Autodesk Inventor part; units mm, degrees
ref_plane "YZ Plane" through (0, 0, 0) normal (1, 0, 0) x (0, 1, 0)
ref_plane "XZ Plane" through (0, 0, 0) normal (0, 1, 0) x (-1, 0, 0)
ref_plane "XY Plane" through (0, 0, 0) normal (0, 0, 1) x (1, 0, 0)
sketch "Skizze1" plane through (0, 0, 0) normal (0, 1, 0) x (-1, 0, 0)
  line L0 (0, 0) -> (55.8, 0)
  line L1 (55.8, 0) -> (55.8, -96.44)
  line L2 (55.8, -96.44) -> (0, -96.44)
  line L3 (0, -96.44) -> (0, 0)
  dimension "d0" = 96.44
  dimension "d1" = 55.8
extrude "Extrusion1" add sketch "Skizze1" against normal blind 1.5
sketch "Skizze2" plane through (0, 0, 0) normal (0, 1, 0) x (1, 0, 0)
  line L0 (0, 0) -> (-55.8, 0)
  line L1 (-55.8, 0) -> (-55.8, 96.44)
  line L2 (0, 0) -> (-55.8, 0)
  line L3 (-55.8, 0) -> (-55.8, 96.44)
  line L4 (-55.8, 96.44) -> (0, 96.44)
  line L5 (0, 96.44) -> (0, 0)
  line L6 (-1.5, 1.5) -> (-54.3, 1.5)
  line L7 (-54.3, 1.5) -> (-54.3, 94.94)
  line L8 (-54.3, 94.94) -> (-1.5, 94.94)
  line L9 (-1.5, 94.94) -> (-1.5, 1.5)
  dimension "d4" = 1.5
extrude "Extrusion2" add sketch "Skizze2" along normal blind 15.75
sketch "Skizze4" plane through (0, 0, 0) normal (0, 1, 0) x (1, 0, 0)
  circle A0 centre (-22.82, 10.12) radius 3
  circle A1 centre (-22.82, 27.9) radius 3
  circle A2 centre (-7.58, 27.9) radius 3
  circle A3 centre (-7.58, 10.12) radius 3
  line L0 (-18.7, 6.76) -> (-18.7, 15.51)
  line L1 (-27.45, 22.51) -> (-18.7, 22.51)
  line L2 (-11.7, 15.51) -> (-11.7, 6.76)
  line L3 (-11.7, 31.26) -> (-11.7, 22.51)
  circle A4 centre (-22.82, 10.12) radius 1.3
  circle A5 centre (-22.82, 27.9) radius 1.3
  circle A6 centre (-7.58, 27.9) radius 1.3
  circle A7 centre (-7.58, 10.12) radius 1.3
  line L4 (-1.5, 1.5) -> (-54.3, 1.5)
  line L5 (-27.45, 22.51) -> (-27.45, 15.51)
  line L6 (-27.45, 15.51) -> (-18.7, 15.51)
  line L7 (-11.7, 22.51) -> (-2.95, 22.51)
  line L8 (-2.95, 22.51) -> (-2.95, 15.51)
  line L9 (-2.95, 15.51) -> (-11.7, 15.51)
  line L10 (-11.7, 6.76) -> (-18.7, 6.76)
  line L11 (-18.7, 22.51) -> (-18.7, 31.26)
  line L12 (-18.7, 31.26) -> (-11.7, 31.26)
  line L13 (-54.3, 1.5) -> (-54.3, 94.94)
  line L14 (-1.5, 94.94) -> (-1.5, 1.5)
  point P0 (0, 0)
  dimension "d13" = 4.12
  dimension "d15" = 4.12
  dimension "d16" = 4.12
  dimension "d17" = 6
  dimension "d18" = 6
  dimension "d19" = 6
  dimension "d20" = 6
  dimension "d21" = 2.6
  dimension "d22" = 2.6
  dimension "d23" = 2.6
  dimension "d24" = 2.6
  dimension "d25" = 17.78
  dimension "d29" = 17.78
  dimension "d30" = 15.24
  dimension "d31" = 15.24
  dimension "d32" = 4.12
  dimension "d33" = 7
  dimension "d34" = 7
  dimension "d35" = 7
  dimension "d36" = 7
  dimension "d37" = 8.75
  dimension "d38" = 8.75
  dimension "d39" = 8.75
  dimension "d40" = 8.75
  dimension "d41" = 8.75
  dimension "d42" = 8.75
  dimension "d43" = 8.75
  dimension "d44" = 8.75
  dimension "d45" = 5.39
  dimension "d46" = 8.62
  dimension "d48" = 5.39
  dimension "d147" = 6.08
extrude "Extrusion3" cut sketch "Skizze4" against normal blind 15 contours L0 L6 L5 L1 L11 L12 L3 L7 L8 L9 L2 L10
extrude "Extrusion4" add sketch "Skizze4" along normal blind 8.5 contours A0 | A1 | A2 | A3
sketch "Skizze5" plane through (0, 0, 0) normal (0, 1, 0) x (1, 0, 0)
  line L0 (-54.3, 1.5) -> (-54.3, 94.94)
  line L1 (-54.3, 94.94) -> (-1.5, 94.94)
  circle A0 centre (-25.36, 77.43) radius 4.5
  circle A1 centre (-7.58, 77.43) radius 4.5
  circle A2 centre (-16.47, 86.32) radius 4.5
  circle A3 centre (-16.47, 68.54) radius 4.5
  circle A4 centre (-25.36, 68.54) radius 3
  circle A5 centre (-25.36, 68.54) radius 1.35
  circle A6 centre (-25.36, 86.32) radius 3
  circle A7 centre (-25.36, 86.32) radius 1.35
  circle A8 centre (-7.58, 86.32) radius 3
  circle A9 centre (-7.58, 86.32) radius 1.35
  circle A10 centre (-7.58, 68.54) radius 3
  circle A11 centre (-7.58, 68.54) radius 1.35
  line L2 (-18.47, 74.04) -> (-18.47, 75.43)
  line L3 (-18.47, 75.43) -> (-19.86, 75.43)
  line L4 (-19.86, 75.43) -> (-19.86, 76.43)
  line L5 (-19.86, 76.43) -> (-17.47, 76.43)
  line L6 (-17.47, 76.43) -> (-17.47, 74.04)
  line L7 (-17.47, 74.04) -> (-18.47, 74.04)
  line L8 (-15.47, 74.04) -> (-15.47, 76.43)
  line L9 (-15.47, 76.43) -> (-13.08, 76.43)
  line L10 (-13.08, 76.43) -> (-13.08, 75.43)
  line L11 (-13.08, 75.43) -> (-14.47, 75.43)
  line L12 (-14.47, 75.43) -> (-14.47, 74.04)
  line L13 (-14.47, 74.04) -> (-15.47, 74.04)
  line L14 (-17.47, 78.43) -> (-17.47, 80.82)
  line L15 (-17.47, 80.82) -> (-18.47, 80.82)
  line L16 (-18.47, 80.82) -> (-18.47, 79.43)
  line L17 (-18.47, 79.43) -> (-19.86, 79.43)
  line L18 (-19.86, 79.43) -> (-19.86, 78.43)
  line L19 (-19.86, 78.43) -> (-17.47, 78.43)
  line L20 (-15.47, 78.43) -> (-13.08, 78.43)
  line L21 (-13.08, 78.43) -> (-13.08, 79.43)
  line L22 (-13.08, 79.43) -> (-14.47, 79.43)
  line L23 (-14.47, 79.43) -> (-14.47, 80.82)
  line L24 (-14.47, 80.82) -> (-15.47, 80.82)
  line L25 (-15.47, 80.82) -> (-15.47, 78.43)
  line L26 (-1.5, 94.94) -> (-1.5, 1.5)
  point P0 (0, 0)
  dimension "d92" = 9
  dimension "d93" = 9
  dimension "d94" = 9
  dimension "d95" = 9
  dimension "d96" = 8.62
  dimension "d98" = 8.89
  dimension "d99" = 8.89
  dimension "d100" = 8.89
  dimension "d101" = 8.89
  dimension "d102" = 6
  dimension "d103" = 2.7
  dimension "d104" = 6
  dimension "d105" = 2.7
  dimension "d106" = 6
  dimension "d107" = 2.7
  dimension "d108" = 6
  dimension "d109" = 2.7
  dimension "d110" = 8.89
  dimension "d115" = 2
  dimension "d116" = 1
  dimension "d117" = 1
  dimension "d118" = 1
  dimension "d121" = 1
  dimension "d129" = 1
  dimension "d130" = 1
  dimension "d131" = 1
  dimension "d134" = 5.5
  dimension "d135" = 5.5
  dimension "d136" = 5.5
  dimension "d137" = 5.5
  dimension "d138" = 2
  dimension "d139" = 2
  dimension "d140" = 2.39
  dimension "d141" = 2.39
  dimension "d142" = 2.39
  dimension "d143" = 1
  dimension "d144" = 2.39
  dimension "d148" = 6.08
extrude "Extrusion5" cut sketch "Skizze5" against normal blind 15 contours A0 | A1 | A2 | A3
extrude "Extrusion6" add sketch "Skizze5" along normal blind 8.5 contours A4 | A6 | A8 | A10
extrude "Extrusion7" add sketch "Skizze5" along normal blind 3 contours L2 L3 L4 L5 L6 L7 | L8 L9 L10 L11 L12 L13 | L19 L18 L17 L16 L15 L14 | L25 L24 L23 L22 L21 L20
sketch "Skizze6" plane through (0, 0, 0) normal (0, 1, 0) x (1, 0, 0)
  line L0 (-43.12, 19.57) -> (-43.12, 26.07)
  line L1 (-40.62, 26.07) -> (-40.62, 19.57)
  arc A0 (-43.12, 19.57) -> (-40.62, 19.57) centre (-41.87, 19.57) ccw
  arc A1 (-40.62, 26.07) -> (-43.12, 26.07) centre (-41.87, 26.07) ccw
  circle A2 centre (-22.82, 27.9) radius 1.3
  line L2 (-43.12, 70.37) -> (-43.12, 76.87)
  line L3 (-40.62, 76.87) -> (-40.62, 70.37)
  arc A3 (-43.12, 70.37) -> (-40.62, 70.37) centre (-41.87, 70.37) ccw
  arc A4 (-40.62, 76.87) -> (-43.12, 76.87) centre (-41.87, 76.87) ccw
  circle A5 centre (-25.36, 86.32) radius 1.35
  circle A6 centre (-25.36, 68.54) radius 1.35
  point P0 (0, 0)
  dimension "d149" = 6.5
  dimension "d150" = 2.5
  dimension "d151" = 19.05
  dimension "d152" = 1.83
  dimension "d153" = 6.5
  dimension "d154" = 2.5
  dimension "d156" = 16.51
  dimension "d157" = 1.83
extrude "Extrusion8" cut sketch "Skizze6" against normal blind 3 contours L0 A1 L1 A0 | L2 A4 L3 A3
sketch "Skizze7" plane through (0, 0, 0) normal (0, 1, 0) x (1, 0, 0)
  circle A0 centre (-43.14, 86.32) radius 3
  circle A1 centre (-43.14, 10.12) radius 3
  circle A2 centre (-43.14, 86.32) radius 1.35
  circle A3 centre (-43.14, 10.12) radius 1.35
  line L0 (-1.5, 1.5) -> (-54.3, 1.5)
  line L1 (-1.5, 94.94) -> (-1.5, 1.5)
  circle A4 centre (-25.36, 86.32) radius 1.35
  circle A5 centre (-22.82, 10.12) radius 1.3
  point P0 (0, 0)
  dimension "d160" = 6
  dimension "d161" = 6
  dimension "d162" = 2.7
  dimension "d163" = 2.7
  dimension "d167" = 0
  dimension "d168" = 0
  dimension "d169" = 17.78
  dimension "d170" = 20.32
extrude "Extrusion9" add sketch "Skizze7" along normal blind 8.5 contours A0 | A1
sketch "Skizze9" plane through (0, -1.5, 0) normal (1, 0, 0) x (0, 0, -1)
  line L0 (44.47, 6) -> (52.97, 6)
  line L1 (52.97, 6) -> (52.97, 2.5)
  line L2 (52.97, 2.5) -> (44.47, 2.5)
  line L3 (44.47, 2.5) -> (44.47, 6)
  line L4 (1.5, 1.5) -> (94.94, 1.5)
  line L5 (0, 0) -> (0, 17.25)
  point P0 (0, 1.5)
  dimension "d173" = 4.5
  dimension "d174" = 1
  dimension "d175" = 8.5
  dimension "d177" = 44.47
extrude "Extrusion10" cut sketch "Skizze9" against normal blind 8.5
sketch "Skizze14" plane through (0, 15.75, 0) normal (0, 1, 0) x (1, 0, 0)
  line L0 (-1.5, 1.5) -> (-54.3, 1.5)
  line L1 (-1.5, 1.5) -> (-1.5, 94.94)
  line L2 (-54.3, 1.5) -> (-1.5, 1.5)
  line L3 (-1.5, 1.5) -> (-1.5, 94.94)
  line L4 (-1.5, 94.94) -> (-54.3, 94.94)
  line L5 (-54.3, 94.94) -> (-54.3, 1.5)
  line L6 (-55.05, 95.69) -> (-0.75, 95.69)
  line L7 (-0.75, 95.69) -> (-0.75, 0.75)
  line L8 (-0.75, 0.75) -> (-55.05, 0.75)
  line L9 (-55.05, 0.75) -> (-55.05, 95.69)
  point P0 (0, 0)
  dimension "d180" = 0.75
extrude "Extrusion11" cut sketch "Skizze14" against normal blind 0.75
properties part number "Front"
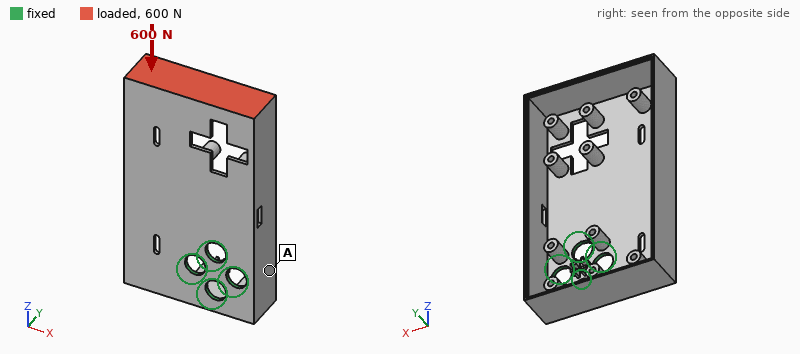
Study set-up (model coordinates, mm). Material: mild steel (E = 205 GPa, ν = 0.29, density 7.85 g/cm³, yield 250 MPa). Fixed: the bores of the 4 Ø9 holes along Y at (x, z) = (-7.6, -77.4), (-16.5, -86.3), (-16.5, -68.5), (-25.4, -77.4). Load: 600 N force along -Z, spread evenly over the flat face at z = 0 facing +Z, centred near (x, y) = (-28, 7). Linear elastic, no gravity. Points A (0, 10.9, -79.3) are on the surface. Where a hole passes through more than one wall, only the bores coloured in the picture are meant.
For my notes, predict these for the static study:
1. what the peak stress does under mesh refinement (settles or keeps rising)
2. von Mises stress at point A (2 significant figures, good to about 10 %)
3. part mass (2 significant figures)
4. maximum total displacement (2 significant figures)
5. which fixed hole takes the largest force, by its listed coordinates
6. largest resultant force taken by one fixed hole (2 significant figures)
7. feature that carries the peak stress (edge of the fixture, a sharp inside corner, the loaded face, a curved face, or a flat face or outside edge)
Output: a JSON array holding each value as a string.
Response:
["keeps rising", "13 MPa", "130 g", "0.35 mm", "(-25.4, -77.4)", "400 N", "a sharp inside corner"]
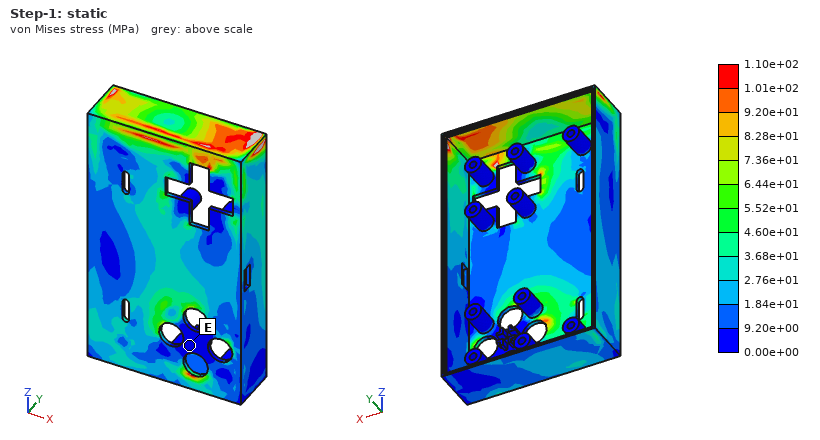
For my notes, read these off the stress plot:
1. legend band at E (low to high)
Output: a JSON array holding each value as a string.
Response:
["0.00e+00 to 9.20e+00 MPa"]
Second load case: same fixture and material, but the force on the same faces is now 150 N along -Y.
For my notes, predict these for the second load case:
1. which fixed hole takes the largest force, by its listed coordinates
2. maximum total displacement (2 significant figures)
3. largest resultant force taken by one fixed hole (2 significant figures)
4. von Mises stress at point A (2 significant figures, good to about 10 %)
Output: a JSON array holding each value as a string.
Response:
["(-16.5, -86.3)", "0.97 mm", "370 N", "27 MPa"]
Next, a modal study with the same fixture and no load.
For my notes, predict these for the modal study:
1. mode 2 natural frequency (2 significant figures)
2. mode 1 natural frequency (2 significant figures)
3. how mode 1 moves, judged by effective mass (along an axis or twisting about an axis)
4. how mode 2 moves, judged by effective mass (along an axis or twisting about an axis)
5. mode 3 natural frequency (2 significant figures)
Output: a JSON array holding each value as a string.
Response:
["930 Hz", "350 Hz", "along Y", "along Y", "1800 Hz"]
